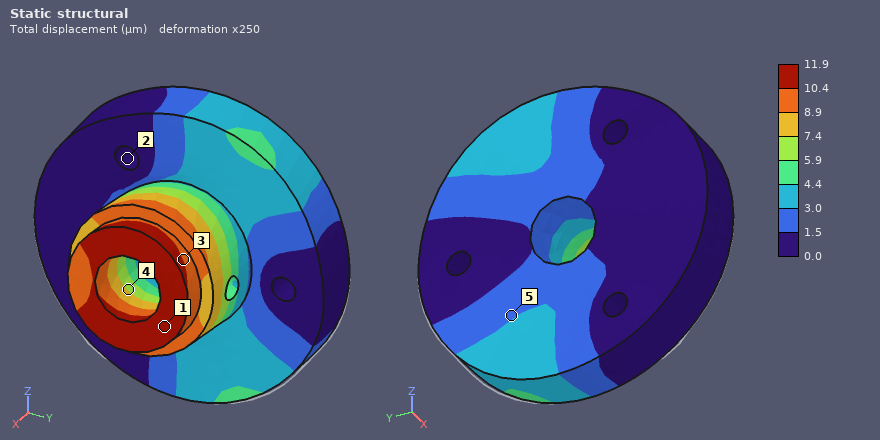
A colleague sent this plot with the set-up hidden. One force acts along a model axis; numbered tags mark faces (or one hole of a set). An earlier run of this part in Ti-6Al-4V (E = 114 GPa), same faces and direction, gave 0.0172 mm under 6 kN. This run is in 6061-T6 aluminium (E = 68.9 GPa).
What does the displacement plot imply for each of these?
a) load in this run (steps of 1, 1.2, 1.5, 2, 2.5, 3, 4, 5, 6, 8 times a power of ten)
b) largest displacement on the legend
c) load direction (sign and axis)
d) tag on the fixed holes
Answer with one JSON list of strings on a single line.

["2.5 kN", "11.9 µm", "+Z", "2"]
